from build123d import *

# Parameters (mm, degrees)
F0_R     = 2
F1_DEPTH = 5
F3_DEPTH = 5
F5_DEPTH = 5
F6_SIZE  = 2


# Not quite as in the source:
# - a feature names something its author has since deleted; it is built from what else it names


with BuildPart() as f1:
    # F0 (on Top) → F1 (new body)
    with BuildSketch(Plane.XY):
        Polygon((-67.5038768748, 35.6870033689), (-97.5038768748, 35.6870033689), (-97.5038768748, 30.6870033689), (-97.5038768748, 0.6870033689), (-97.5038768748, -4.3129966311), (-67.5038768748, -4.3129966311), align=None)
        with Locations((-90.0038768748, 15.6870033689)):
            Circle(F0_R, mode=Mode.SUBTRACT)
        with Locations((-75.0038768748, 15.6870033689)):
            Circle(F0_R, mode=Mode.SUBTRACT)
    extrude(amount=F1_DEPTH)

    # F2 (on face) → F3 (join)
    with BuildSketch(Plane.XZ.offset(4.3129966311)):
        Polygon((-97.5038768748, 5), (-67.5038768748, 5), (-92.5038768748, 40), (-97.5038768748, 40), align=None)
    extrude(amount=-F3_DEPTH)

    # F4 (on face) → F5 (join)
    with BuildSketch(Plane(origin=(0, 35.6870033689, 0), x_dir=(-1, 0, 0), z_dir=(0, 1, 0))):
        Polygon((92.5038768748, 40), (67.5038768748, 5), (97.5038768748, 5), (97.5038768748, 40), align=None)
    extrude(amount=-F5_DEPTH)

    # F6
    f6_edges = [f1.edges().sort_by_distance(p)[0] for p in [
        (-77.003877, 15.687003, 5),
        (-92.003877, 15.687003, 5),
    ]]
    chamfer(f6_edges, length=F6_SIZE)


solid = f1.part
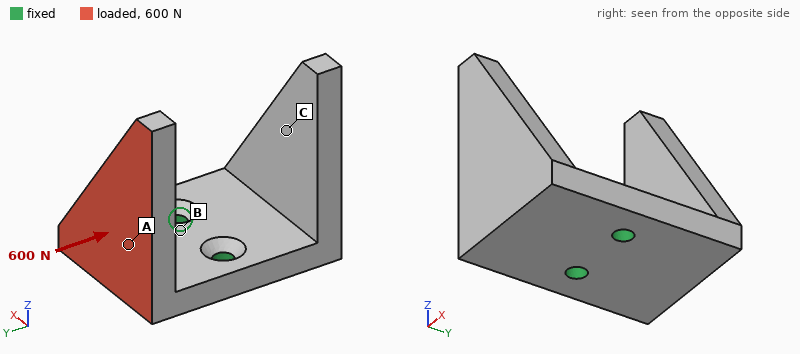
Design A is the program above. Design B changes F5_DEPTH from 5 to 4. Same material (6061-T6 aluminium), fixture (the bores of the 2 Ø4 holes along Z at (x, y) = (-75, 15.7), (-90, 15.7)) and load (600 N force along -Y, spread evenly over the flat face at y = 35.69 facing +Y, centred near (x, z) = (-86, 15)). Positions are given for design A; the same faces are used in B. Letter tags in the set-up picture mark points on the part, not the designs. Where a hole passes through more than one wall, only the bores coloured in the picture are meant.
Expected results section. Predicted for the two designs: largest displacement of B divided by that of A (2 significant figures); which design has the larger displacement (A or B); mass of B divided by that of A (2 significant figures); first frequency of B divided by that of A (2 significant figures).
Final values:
1.3
B
0.95
1.0
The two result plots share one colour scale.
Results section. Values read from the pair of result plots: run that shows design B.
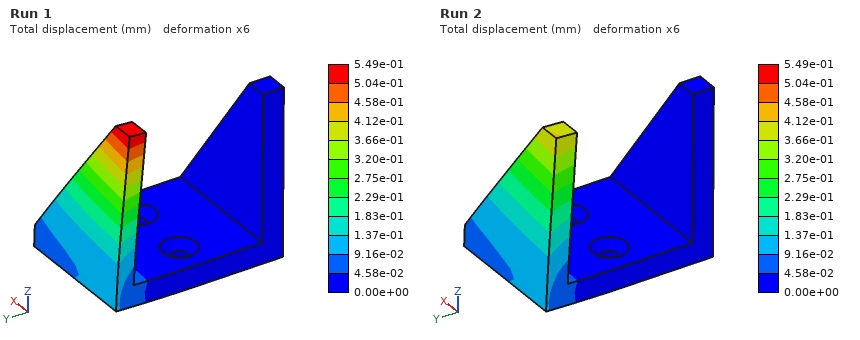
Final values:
Run 1
